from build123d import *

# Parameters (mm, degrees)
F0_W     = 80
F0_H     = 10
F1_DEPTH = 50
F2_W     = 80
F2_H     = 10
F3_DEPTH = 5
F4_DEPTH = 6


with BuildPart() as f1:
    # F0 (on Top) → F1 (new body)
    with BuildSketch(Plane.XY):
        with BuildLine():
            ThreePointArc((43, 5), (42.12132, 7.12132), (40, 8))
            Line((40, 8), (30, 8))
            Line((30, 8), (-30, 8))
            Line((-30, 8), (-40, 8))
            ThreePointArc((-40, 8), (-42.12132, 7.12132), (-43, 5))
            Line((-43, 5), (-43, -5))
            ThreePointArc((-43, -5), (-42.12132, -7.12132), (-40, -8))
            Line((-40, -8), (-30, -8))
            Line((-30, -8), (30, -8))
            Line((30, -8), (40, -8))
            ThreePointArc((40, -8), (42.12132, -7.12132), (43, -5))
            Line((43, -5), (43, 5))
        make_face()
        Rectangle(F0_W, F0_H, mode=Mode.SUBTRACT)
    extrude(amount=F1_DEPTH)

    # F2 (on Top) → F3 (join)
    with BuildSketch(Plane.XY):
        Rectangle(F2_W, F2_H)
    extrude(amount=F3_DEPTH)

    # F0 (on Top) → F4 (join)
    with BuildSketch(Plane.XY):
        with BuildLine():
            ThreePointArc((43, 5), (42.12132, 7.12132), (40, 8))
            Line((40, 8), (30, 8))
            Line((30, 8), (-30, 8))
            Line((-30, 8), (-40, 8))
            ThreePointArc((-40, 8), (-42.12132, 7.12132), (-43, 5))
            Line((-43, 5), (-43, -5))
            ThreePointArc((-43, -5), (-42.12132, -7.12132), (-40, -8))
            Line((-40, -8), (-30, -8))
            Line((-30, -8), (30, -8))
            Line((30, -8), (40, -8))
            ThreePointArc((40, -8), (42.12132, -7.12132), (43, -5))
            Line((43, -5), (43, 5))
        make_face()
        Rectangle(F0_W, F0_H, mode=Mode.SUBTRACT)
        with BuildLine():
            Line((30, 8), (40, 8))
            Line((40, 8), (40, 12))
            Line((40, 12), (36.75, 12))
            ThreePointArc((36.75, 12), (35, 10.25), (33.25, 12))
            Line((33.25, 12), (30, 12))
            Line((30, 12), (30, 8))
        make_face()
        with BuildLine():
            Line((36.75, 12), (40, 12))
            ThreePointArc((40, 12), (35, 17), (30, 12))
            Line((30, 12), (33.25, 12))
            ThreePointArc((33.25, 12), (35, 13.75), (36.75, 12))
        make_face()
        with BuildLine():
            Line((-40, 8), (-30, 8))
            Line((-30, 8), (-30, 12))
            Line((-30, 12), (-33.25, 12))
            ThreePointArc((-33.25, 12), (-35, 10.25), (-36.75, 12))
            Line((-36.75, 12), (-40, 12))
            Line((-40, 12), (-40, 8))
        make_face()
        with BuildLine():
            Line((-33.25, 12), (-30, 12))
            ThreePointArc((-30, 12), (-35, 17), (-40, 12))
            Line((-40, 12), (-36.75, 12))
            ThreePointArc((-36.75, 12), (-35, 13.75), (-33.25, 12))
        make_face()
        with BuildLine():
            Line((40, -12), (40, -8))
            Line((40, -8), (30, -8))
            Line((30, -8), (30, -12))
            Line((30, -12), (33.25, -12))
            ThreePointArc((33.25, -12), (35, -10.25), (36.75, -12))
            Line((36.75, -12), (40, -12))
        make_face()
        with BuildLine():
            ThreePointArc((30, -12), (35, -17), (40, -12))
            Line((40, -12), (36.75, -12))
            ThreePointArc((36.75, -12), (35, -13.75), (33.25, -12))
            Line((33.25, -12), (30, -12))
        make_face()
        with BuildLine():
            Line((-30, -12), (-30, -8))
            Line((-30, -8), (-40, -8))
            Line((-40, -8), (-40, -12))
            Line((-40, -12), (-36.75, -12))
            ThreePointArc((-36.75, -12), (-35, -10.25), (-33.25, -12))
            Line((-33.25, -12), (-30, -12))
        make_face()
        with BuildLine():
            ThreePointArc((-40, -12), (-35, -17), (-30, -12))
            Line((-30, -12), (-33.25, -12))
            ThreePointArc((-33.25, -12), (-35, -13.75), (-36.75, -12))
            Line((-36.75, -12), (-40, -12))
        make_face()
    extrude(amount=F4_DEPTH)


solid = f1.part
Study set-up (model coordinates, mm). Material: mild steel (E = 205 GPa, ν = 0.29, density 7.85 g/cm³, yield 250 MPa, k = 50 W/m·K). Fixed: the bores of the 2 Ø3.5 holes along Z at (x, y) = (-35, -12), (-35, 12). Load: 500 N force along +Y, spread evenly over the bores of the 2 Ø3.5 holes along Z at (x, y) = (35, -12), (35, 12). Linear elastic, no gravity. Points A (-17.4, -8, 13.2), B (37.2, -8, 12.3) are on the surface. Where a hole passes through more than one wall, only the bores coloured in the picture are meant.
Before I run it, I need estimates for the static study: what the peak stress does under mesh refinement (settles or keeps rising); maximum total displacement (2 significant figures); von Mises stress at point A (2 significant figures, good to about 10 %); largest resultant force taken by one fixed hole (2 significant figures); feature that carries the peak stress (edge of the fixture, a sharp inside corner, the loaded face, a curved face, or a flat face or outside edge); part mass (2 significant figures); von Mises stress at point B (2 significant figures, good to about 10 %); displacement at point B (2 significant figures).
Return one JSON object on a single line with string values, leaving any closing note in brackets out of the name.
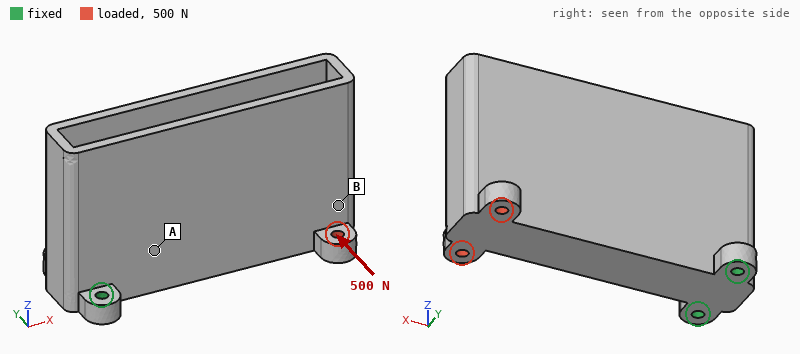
{"what the peak stress does under mesh refinement": "keeps rising", "maximum total displacement": "95 µm", "von Mises stress at point A": "30 MPa", "largest resultant force taken by one fixed hole": "1.7 kN", "feature that carries the peak stress": "edge of the fixture", "part mass": "270 g", "von Mises stress at point B": "8.6 MPa", "displacement at point B": "82 µm"}
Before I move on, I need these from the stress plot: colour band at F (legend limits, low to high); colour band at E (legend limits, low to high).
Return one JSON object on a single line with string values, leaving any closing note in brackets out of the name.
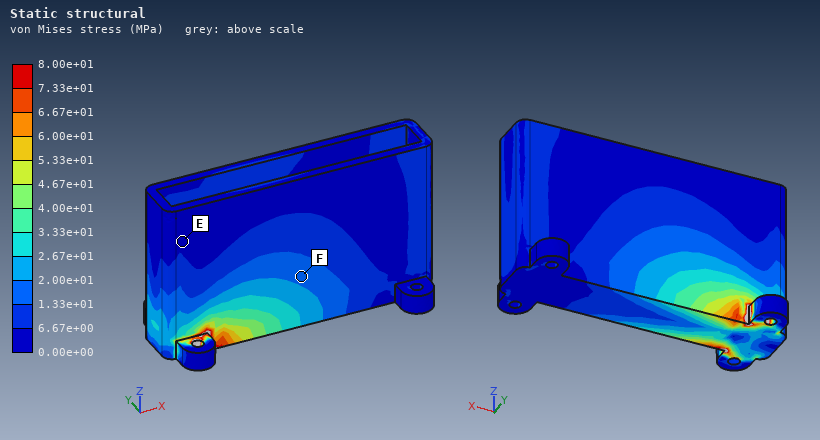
{"colour band at F": "1.33e+01 to 2.00e+01 MPa", "colour band at E": "0.00e+00 to 6.67e+00 MPa"}
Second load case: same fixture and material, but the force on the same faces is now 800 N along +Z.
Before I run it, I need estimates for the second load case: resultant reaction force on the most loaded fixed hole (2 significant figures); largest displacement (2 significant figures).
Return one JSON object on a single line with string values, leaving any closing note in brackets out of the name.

{"resultant reaction force on the most loaded fixed hole": "420 N", "largest displacement": "0.38 mm"}
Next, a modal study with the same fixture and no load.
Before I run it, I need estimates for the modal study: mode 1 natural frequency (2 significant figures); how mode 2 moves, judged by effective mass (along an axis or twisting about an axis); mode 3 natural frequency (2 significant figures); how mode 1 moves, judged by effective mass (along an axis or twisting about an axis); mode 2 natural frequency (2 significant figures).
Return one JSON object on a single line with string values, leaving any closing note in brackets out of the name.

{"mode 1 natural frequency": "710 Hz", "how mode 2 moves, judged by effective mass": "along Y", "mode 3 natural frequency": "2400 Hz", "how mode 1 moves, judged by effective mass": "along Z", "mode 2 natural frequency": "930 Hz"}
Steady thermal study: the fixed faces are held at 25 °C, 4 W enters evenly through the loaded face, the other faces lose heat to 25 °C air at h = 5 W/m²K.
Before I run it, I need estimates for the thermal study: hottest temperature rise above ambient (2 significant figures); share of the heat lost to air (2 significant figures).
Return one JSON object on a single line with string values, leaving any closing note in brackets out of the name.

{"hottest temperature rise above ambient": "26 K", "share of the heat lost to air": "29 %"}
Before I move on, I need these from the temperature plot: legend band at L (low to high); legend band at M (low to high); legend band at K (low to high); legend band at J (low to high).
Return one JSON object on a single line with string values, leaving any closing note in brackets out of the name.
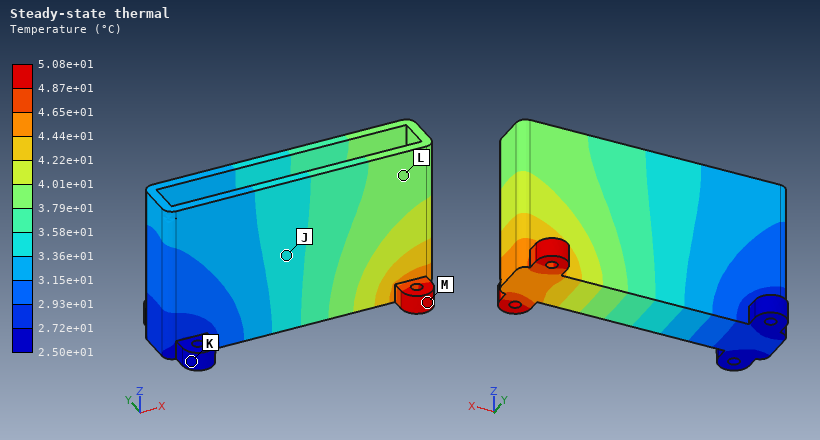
{"legend band at L": "3.79e+01 to 4.01e+01 °C", "legend band at M": "4.87e+01 to 5.08e+01 °C", "legend band at K": "2.50e+01 to 2.72e+01 °C", "legend band at J": "3.36e+01 to 3.58e+01 °C"}
